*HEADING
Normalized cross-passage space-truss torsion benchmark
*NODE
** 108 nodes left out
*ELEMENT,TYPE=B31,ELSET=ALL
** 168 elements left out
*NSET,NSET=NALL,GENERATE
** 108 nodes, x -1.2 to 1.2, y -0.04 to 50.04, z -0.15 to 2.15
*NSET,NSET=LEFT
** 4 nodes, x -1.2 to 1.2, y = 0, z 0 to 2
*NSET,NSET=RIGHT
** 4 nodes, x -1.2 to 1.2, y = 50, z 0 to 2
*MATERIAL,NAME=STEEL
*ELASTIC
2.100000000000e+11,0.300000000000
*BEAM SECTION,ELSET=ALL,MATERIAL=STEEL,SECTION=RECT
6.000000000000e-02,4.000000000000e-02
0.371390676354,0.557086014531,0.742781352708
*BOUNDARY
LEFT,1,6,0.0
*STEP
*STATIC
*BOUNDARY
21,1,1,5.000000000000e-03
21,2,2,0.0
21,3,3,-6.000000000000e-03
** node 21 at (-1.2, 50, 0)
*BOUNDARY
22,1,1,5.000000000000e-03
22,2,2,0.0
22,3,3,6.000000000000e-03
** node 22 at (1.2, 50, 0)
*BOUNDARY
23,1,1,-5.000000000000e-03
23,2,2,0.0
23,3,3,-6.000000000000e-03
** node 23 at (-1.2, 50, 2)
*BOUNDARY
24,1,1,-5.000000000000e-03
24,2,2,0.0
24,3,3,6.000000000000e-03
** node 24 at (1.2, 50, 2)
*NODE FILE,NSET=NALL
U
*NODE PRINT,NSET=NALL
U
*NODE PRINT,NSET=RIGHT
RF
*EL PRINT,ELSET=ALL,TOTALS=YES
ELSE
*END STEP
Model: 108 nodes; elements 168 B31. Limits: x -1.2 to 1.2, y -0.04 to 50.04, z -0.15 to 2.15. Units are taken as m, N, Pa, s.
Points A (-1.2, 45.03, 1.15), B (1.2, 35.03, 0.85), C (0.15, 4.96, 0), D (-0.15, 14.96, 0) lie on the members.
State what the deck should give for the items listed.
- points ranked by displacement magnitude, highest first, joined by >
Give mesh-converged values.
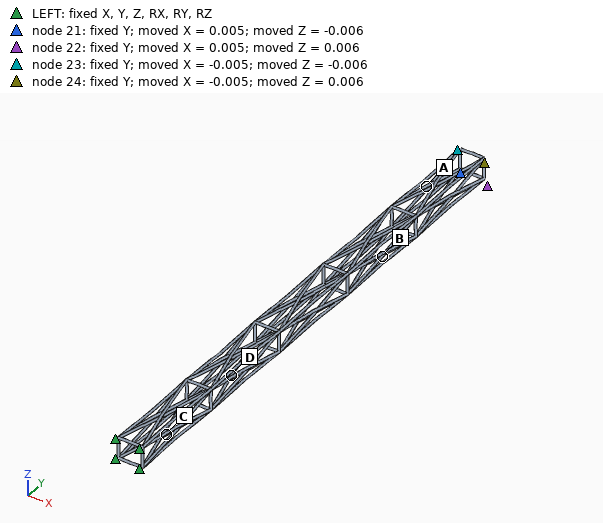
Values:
A > B > C > D
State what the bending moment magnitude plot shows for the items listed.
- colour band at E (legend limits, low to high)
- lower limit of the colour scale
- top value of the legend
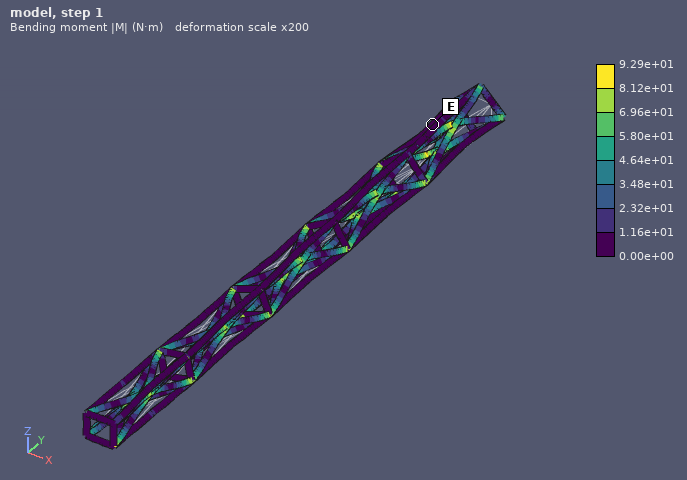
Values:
0.00e+00 to 1.16e+01 N·m
0.00e+00 N·m
9.29e+01 N·m
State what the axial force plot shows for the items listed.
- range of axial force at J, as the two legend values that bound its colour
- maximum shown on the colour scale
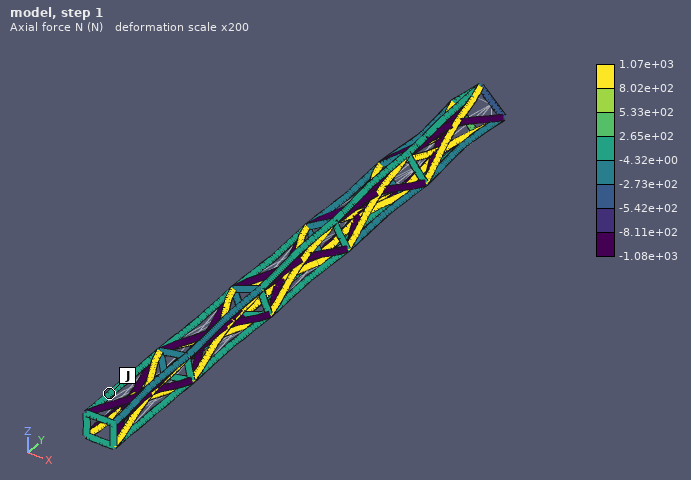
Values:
-4.32e+00 to 2.65e+02 N
1.07e+03 N
